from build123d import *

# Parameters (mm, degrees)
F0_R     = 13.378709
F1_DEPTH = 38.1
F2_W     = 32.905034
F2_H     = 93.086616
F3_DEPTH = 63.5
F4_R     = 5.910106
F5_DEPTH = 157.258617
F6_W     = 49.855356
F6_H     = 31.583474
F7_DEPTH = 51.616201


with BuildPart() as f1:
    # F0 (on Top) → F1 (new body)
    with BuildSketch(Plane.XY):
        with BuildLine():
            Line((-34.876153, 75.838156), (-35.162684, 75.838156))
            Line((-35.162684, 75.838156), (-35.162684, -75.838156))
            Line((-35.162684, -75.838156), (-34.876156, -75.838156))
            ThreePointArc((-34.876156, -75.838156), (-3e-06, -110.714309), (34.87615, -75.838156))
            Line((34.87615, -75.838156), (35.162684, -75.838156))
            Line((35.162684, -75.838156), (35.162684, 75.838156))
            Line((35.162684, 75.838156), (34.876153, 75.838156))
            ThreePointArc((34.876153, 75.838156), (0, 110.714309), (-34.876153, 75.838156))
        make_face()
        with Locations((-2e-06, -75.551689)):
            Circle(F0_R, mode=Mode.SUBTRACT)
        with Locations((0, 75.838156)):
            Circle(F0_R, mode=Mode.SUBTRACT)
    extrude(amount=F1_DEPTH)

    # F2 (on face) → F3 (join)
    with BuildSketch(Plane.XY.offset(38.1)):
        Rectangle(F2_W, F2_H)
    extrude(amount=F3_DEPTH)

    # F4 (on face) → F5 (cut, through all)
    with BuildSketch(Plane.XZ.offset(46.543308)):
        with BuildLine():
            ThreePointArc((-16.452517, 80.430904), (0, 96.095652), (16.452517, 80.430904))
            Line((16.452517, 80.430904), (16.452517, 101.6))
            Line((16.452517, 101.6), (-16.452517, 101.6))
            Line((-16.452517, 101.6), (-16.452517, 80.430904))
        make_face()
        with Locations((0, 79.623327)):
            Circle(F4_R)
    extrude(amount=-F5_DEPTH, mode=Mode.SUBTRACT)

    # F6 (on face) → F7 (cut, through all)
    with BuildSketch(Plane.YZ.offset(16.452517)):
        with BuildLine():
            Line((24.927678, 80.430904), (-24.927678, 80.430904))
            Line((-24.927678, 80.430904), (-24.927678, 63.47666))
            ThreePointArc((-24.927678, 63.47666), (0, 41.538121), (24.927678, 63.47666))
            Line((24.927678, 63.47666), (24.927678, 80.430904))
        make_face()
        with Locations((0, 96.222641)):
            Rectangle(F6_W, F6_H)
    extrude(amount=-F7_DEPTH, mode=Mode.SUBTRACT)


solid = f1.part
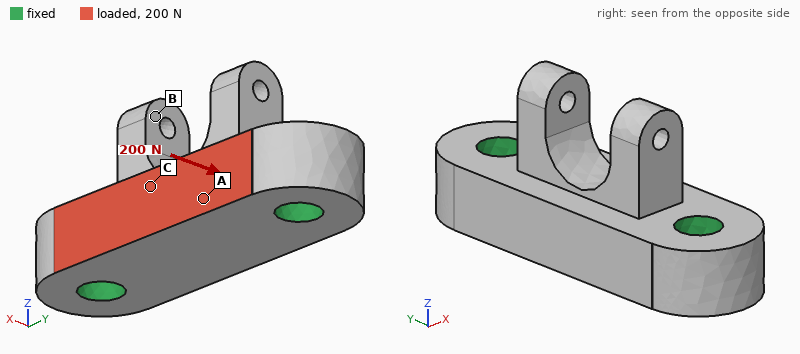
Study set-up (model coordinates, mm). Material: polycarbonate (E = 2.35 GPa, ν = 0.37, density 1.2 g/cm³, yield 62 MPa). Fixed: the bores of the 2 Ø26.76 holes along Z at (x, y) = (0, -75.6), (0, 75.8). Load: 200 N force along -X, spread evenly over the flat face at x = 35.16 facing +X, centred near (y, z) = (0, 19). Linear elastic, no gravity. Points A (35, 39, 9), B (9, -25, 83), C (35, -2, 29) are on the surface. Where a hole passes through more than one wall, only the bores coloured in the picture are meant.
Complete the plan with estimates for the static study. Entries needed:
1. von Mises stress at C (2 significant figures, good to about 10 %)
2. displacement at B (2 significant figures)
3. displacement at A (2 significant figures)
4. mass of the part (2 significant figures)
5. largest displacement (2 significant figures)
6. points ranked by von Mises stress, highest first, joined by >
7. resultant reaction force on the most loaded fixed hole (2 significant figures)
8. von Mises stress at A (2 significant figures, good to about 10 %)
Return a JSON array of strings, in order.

["0.063 MPa", "2.3 µm", "2.0 µm", "720 g", "2.9 µm", "C > A > B", "100 N", "0.038 MPa"]
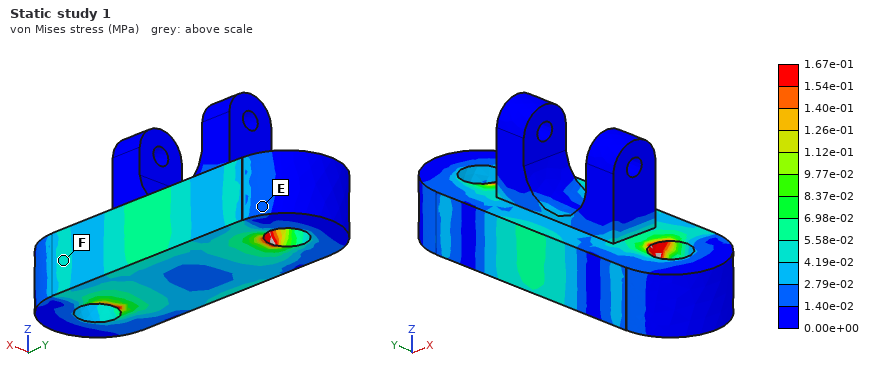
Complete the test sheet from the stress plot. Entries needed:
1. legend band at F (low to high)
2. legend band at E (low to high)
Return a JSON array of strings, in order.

["4.19e-02 to 5.58e-02 MPa", "1.40e-02 to 2.79e-02 MPa"]
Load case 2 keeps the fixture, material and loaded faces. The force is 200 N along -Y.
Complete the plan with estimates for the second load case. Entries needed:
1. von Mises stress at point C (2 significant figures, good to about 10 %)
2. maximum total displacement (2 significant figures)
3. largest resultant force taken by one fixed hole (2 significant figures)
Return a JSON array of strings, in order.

["0.061 MPa", "1.5 µm", "110 N"]
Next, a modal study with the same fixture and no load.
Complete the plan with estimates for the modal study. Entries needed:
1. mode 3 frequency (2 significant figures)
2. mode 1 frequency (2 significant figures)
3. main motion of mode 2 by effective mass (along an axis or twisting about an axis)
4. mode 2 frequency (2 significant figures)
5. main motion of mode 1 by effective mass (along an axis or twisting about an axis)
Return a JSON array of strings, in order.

["1800 Hz", "1400 Hz", "along Z", "1600 Hz", "along X"]
